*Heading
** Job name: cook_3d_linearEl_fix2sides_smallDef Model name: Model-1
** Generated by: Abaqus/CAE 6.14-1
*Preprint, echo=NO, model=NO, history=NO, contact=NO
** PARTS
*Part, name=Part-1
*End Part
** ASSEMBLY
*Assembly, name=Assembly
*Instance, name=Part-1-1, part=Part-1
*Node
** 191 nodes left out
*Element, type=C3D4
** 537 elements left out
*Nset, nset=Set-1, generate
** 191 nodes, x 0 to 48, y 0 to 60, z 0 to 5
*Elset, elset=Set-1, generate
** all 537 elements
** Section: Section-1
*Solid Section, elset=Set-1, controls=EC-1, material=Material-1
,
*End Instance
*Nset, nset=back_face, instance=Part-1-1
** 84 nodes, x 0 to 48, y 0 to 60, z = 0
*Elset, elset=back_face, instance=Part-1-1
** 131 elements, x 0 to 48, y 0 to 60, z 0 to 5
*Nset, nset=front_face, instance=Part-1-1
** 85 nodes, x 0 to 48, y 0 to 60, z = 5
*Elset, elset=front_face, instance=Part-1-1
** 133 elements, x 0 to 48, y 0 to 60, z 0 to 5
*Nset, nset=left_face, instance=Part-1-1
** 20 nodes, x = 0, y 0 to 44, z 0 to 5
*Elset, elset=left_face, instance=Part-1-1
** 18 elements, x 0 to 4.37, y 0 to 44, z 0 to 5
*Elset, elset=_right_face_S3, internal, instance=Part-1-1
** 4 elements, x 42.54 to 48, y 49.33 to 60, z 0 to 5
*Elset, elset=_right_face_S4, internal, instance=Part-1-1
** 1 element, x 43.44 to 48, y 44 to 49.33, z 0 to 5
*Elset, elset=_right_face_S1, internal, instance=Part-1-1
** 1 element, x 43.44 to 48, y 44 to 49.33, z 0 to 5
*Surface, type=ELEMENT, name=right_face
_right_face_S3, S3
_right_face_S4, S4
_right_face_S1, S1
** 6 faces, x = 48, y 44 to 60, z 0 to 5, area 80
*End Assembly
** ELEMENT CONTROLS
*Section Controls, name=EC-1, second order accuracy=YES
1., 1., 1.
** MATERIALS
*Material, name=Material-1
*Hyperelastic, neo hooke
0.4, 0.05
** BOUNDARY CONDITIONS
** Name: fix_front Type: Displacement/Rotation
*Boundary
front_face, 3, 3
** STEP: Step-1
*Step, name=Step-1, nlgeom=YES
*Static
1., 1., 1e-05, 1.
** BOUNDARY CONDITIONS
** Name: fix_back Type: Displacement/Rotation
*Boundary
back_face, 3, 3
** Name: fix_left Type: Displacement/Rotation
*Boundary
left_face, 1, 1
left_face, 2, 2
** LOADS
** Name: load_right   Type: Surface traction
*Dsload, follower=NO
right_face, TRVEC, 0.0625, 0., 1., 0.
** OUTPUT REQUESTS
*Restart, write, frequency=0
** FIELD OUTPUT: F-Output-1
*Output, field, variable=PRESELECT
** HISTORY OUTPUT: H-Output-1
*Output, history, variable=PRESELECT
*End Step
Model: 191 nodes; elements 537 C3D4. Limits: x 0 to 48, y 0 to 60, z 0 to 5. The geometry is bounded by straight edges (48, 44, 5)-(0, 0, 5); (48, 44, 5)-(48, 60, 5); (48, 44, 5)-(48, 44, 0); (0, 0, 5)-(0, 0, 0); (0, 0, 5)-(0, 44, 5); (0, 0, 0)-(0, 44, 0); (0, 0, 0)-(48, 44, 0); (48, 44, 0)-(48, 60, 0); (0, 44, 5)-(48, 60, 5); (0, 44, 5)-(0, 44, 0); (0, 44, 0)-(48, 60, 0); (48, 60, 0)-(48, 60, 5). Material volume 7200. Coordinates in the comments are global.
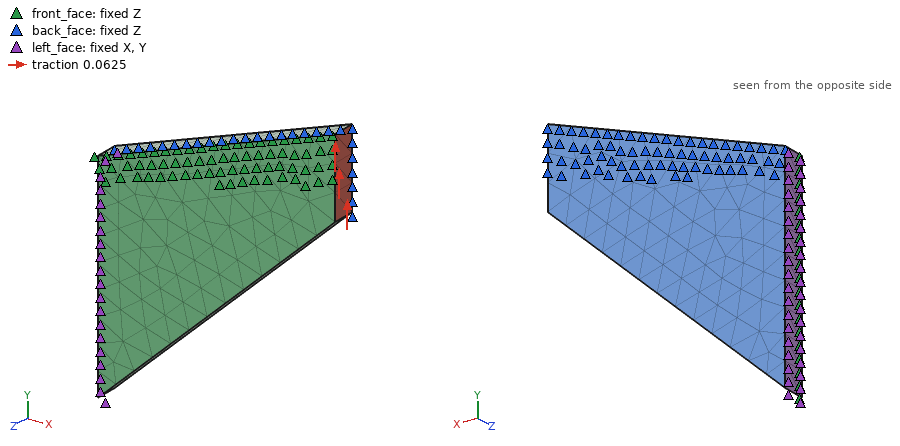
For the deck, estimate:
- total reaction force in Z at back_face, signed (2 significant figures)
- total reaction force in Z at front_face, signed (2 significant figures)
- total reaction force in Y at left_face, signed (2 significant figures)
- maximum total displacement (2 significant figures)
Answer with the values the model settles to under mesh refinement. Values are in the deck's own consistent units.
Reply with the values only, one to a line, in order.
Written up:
-21
21
-5.0
9.2
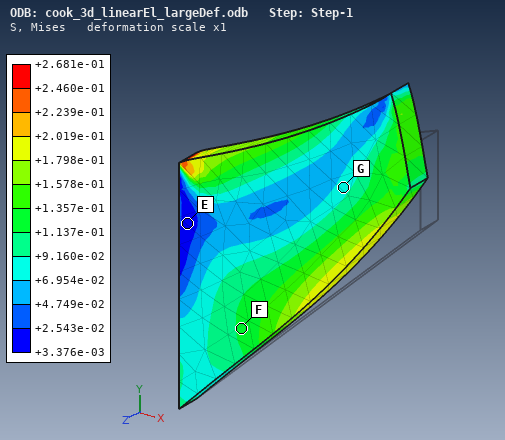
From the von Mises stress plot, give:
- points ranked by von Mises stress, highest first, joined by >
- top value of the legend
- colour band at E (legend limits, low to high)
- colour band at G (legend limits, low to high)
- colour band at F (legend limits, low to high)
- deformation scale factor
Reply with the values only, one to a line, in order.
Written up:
F > G > E
+2.681e-01
+3.376e-03 to +2.543e-02
+6.954e-02 to +9.160e-02
+1.137e-01 to +1.357e-01
1
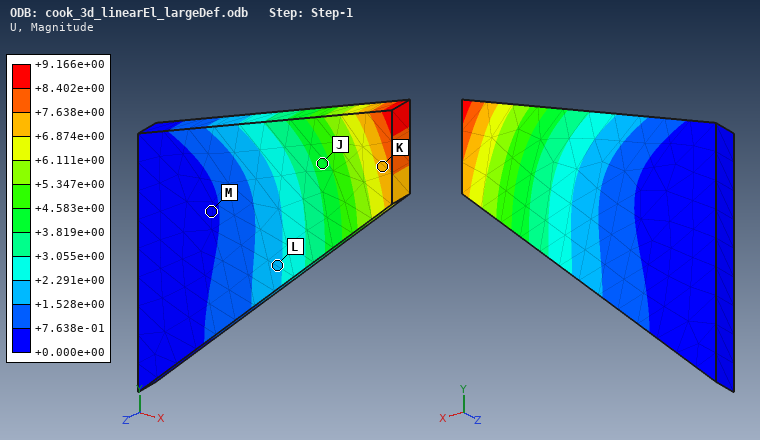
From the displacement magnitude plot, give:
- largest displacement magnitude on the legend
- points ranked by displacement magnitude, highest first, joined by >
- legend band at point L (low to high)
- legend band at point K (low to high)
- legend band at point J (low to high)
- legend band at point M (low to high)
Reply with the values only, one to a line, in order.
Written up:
+9.166e+00
K > J > L > M
+1.528e+00 to +2.291e+00
+6.874e+00 to +7.638e+00
+3.819e+00 to +4.583e+00
+0.000e+00 to +7.638e-01
